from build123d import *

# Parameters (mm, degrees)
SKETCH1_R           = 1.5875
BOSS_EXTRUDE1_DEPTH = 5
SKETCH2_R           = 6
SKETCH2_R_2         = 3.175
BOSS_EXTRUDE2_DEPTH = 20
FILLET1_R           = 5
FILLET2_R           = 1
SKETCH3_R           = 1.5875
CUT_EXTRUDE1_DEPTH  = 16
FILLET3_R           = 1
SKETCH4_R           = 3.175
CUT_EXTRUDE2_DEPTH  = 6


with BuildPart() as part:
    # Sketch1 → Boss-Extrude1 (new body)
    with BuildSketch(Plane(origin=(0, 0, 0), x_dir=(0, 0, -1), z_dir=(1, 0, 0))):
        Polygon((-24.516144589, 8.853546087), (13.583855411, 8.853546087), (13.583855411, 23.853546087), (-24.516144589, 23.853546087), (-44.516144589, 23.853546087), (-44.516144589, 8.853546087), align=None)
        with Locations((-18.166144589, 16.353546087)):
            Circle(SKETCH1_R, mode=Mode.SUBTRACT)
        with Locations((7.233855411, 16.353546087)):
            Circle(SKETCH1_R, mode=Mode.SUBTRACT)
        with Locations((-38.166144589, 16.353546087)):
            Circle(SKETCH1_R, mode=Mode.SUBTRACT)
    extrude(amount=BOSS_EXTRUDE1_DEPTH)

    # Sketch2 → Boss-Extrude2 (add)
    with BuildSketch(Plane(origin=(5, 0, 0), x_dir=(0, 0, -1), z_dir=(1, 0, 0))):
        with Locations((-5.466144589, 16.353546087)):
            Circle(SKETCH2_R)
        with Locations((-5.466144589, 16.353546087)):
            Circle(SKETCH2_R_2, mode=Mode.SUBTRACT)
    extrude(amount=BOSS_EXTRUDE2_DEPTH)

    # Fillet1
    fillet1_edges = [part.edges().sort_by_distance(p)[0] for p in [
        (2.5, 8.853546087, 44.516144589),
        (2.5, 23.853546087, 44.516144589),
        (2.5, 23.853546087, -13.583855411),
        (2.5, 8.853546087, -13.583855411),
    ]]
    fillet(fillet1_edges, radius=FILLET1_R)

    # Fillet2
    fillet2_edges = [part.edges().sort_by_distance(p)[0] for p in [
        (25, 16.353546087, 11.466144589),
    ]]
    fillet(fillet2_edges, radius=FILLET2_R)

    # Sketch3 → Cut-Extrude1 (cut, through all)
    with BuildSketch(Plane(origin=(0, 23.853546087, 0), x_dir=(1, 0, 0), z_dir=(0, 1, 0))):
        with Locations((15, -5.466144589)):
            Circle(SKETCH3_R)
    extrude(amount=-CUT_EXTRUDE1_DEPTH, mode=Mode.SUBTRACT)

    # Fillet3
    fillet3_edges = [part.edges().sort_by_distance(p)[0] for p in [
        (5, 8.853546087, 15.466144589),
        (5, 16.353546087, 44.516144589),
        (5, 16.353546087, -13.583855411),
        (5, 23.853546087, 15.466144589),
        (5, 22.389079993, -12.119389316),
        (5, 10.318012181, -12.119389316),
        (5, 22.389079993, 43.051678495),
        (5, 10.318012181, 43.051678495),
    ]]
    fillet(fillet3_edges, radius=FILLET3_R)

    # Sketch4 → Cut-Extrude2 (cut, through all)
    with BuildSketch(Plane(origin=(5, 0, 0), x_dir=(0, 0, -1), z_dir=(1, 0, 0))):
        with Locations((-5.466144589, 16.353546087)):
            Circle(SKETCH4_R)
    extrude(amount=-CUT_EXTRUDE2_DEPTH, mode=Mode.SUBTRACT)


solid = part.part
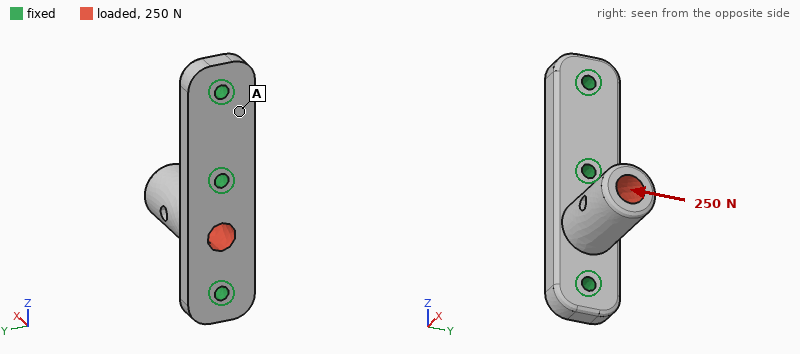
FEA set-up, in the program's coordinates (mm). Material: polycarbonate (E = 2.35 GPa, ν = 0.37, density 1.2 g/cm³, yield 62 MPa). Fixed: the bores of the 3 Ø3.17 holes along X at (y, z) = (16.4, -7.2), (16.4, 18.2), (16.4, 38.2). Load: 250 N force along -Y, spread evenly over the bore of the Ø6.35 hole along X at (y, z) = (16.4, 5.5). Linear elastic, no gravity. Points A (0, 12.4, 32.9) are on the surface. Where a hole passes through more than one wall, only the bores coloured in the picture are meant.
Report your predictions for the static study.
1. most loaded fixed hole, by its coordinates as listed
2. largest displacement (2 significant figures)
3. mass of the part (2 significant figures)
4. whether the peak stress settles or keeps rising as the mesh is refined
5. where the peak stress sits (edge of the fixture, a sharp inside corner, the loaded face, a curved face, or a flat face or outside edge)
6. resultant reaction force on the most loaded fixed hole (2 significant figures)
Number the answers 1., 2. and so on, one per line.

1. (16.4, 18.2)
2. 0.75 mm
3. 6.6 g
4. keeps rising
5. edge of the fixture
6. 150 N
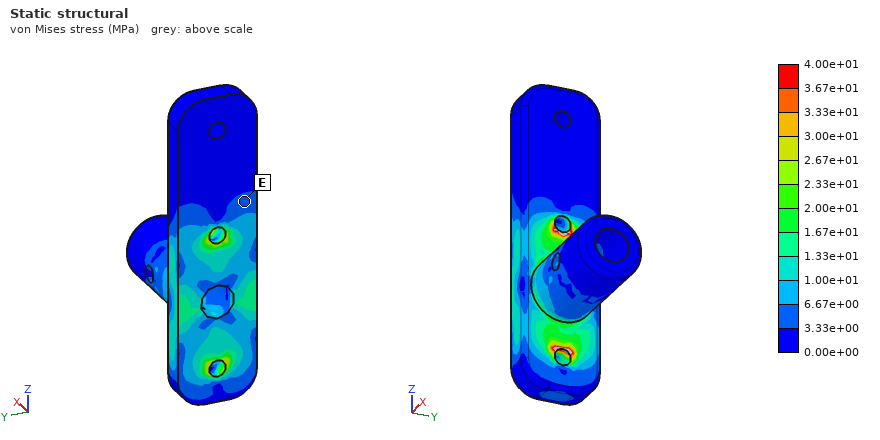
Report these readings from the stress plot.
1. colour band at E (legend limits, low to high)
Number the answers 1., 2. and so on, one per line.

1. 3.33e+00 to 6.67e+00 MPa
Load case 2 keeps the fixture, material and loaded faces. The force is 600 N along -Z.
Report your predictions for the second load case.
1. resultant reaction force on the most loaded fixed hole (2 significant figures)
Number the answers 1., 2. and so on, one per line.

1. 430 N
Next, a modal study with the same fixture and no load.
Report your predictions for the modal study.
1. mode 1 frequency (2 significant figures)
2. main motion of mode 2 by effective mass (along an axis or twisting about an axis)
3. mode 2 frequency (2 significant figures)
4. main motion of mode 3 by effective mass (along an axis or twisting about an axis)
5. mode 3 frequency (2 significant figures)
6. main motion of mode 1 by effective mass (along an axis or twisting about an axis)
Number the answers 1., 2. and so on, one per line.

1. 2200 Hz
2. along Z
3. 3600 Hz
4. along X
5. 6000 Hz
6. along Y
